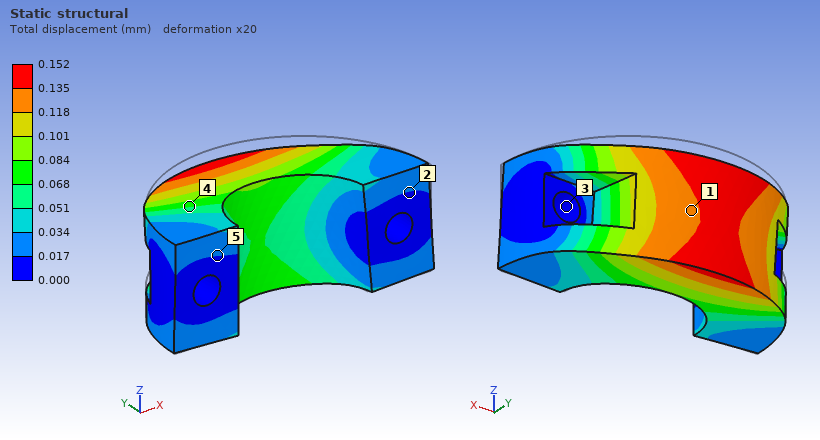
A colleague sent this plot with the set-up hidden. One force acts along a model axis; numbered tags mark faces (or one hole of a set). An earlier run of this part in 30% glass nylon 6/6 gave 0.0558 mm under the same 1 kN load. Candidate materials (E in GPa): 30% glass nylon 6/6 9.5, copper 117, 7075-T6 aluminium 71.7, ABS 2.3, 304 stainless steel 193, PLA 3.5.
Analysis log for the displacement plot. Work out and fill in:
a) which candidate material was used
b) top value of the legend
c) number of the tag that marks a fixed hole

PLA
0.152 mm
3
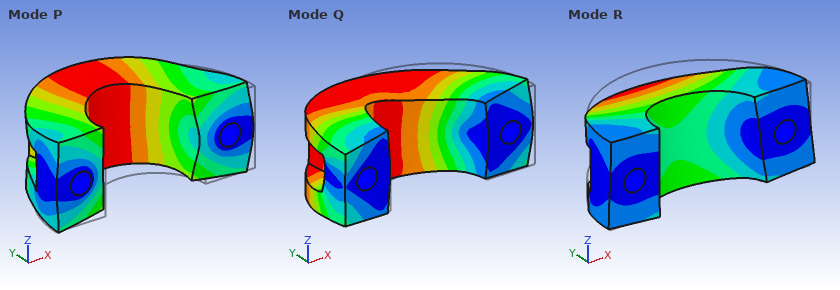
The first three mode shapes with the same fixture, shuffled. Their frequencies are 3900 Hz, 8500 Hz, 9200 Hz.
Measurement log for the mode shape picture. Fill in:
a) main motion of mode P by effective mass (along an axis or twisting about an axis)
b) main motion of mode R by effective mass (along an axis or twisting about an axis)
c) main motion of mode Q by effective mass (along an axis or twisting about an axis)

along Y
along Z
along X
